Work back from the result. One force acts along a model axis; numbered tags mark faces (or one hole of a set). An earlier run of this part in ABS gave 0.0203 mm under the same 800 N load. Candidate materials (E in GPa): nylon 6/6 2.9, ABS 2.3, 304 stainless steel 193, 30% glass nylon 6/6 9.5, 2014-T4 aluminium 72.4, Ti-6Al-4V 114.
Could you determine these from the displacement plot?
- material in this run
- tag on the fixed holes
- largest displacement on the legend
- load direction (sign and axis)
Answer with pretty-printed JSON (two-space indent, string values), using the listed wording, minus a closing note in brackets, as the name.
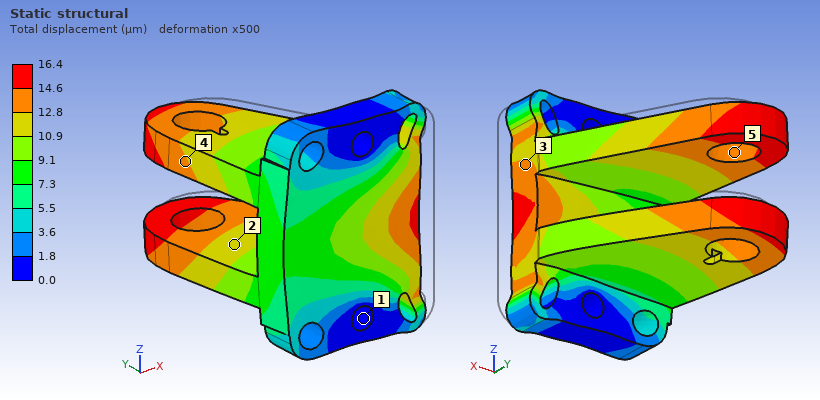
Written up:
{
  "material in this run": "nylon 6/6",
  "tag on the fixed holes": "1",
  "largest displacement on the legend": "16.4 µm",
  "load direction": "-X"
}
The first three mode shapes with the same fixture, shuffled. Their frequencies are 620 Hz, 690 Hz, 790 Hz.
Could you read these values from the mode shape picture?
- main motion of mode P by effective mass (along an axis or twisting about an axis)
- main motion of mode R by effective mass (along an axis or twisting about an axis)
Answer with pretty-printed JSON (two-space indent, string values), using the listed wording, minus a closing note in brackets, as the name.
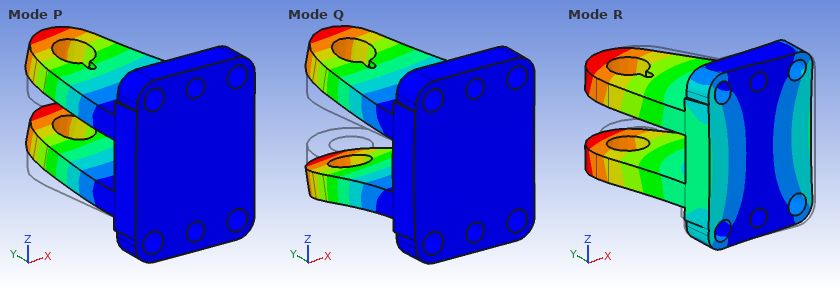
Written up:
{
  "main motion of mode P by effective mass": "along Z",
  "main motion of mode R by effective mass": "along X"
}
